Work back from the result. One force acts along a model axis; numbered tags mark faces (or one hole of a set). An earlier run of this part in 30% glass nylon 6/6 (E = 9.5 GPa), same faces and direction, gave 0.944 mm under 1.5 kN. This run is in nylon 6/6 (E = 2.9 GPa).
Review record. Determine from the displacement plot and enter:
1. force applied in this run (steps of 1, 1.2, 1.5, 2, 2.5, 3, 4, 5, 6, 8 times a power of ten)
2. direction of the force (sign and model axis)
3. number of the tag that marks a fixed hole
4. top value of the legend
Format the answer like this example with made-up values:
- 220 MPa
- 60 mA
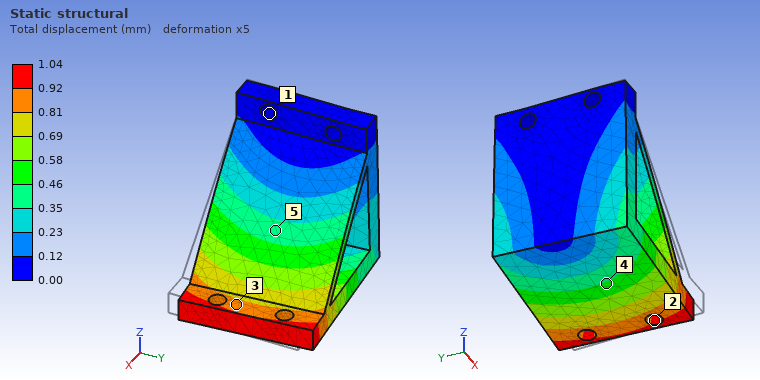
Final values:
- 500 N
- +Y
- 1
- 1.04 mm
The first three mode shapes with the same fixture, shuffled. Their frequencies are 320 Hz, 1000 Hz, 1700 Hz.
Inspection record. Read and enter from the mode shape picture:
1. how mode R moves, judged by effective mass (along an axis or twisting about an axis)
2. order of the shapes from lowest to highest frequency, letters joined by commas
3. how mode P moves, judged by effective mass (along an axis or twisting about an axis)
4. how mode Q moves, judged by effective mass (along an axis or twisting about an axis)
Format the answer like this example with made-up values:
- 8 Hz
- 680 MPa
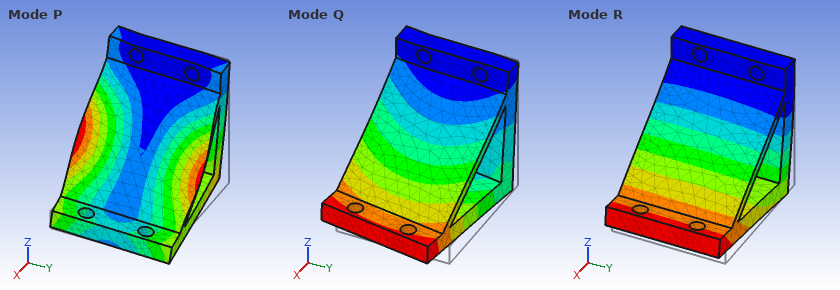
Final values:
- along X
- R, Q, P
- along Y
- along Y
